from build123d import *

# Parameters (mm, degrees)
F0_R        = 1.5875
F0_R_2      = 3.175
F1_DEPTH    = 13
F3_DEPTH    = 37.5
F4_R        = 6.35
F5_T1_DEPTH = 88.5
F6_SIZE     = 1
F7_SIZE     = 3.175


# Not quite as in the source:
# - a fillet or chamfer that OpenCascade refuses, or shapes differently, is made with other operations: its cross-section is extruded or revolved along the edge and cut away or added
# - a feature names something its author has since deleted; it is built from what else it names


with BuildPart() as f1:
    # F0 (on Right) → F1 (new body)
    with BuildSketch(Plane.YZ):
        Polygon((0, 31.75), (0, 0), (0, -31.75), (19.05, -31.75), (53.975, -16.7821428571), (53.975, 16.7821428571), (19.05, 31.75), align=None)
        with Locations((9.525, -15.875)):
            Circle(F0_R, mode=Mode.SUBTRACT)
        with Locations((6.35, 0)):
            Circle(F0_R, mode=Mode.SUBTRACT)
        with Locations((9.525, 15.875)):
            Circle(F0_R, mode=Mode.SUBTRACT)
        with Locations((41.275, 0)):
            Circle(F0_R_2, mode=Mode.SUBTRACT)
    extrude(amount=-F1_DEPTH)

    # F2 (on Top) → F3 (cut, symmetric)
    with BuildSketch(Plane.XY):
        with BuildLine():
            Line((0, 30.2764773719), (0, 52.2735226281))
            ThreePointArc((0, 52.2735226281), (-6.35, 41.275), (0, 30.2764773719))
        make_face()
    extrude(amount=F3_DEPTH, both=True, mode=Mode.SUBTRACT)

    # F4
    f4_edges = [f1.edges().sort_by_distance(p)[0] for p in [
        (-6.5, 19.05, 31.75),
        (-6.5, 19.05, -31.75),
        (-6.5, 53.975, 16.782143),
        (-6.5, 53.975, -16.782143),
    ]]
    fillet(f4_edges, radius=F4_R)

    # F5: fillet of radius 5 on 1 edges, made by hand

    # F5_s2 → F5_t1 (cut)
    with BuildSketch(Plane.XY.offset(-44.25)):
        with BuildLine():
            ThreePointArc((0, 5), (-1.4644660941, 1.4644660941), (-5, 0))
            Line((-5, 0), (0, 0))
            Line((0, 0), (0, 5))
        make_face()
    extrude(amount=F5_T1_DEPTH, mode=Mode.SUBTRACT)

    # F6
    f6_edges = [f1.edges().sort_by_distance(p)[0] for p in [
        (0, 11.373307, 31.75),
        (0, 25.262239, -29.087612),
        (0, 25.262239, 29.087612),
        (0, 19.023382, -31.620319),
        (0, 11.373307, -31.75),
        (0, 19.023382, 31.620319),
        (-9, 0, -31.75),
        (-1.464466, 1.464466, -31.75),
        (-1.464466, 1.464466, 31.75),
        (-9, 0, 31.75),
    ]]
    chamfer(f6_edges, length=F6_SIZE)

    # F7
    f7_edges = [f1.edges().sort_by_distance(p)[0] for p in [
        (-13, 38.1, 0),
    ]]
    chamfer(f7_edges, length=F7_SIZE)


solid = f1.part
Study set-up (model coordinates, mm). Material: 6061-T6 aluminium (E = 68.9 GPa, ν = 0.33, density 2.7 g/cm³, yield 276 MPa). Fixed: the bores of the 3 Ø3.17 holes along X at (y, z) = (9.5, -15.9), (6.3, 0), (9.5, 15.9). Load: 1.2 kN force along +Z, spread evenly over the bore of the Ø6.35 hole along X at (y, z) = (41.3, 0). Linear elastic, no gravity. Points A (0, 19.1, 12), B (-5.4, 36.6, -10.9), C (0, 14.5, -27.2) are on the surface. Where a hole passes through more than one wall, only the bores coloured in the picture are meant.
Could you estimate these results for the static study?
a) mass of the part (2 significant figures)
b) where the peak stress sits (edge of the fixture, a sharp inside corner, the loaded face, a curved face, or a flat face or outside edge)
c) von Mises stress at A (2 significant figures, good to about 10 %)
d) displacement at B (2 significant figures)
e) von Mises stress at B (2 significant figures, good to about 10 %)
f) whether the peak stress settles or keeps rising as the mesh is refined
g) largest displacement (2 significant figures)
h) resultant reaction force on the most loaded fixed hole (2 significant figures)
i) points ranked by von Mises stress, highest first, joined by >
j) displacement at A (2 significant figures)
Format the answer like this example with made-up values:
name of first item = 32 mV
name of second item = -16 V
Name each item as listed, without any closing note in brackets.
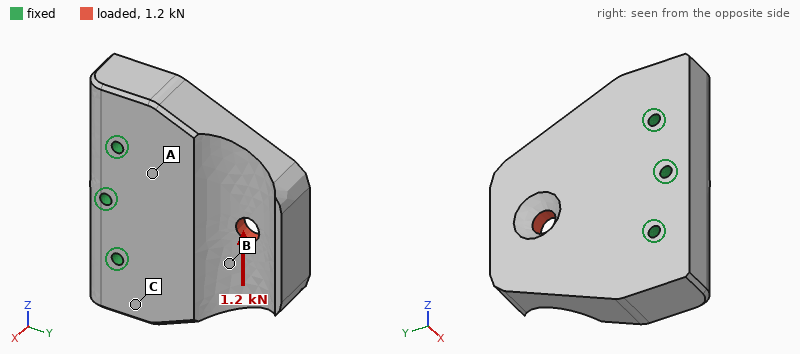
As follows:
mass of the part = 87 g
where the peak stress sits = edge of the fixture
von Mises stress at A = 5.0 MPa
displacement at B = 4.4 µm
von Mises stress at B = 8.7 MPa
whether the peak stress settles or keeps rising as the mesh is refined = keeps rising
largest displacement = 8.0 µm
resultant reaction force on the most loaded fixed hole = 1.3 kN
points ranked by von Mises stress, highest first, joined by > = B > A > C
displacement at A = 1.4 µm
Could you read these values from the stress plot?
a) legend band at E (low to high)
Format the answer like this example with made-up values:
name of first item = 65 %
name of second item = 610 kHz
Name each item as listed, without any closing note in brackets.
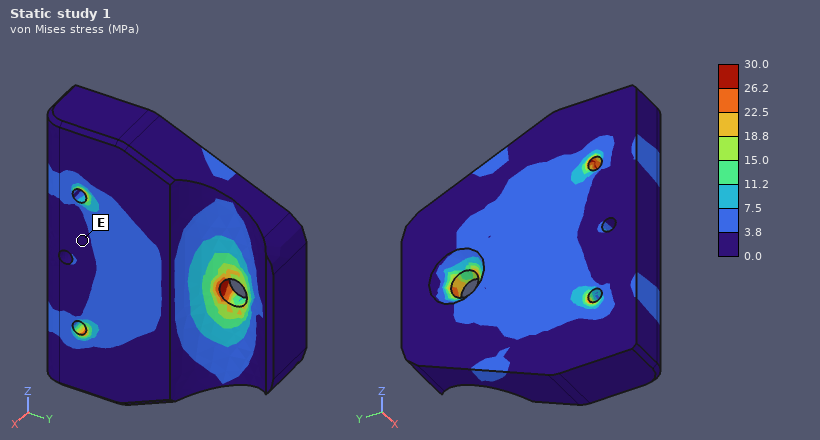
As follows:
legend band at E = 0.0 to 3.8 MPa
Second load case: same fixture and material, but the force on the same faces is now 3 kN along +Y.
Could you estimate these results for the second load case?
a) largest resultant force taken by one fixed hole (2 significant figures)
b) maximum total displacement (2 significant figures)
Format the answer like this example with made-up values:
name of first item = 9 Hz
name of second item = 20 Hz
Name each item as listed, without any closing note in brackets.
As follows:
largest resultant force taken by one fixed hole = 1.1 kN
maximum total displacement = 9.0 µm
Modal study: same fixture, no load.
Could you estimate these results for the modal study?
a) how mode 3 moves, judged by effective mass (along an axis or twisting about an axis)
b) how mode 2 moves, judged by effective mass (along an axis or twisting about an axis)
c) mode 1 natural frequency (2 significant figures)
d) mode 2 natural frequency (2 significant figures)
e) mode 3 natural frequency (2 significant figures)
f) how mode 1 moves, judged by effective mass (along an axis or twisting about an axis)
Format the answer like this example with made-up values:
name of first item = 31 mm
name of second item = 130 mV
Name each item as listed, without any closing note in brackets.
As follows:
how mode 3 moves, judged by effective mass = along Z
how mode 2 moves, judged by effective mass = twisting about Y
mode 1 natural frequency = 5600 Hz
mode 2 natural frequency = 11 kHz
mode 3 natural frequency = 13 kHz
how mode 1 moves, judged by effective mass = along X
